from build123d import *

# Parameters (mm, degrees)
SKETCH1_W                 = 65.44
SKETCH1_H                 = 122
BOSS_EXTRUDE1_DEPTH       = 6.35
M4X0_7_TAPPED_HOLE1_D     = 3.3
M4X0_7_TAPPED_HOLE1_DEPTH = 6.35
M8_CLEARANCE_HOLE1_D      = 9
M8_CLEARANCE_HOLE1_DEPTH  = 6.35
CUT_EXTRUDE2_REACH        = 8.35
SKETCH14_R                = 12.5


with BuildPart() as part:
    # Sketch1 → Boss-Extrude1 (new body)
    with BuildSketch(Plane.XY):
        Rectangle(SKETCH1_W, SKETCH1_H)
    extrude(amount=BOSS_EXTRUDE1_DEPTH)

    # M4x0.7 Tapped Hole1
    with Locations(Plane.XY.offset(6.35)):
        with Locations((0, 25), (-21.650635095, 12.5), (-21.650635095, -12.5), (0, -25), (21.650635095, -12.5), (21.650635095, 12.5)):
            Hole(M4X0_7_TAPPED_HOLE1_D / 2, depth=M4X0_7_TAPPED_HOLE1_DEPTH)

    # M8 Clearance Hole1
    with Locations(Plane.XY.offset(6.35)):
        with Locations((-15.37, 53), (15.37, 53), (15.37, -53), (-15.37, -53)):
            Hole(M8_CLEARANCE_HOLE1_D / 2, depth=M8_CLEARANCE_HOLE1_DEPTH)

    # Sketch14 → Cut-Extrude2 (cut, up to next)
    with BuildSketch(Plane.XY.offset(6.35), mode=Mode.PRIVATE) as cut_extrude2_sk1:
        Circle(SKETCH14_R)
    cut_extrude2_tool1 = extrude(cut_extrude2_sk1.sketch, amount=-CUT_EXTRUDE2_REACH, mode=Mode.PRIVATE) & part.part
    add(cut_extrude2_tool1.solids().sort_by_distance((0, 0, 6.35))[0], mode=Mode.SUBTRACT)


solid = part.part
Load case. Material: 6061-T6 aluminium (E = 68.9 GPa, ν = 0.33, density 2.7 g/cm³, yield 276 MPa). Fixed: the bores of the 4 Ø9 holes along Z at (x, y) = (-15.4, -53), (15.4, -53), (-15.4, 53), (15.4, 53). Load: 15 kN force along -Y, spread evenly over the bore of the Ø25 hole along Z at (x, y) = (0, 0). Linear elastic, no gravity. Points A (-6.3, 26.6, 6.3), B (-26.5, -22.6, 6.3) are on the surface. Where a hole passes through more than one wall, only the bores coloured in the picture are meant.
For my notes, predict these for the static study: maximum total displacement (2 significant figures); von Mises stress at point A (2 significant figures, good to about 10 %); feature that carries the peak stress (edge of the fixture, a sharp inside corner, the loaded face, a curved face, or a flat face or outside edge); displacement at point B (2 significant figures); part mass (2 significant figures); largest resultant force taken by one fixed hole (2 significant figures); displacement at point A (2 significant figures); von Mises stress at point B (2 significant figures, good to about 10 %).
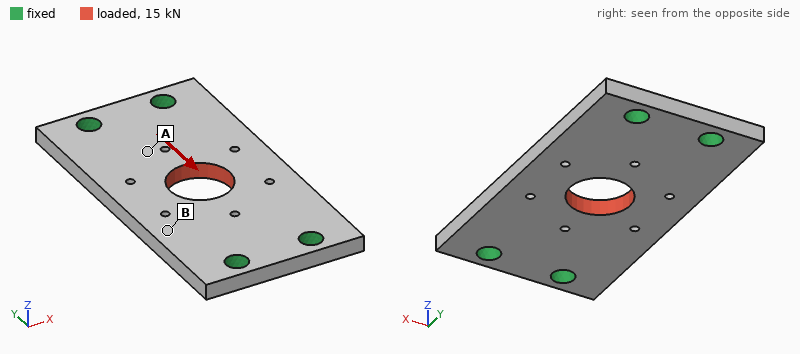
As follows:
18 µm
29 MPa
a curved face
8.9 µm
120 g
3.8 kN
9.6 µm
9.1 MPa
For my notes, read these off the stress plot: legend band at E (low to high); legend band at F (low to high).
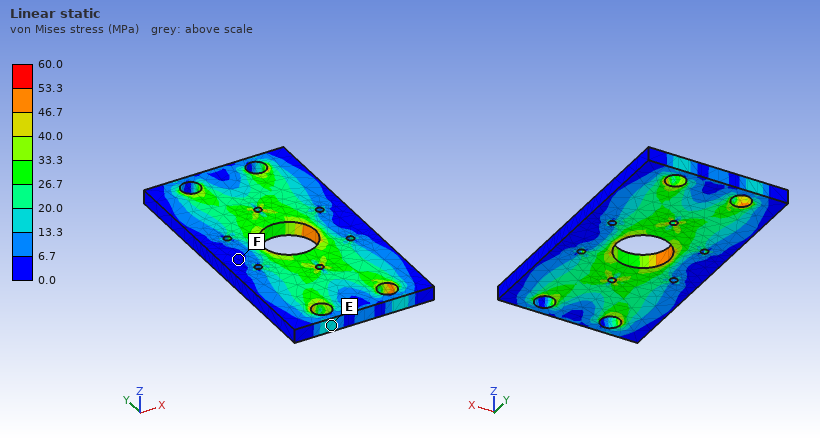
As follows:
13.3 to 20.0 MPa
0.0 to 6.7 MPa
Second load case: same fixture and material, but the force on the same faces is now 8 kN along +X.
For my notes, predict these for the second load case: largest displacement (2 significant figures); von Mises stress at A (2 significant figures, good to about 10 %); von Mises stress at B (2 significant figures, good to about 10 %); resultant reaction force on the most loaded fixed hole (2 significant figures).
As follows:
30 µm
27 MPa
13 MPa
2.8 kN
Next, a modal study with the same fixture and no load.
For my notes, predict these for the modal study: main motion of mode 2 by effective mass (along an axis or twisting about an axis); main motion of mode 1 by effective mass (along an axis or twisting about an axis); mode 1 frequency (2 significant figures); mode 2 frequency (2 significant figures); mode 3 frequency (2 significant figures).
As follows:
twisting about Y
along Z
3200 Hz
4000 Hz
7800 Hz
